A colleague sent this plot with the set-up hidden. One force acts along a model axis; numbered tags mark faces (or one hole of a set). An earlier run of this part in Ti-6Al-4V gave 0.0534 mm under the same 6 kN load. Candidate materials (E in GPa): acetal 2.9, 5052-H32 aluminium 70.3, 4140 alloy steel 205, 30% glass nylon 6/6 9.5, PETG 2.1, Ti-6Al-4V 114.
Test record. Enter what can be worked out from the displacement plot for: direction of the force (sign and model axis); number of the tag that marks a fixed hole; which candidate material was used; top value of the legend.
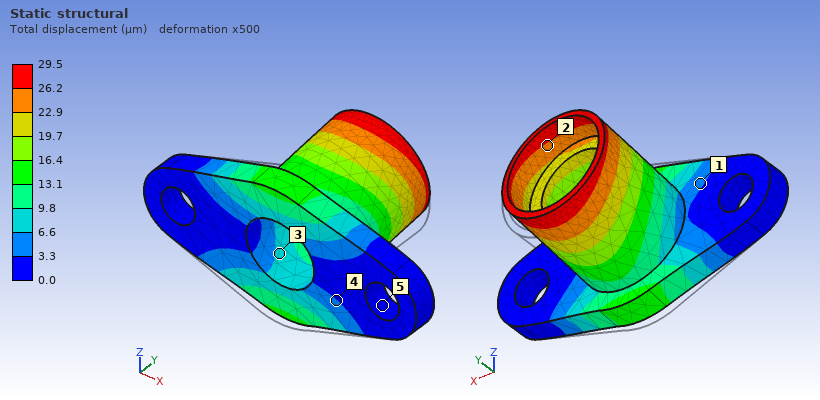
+Z
5
4140 alloy steel
29.5 µm
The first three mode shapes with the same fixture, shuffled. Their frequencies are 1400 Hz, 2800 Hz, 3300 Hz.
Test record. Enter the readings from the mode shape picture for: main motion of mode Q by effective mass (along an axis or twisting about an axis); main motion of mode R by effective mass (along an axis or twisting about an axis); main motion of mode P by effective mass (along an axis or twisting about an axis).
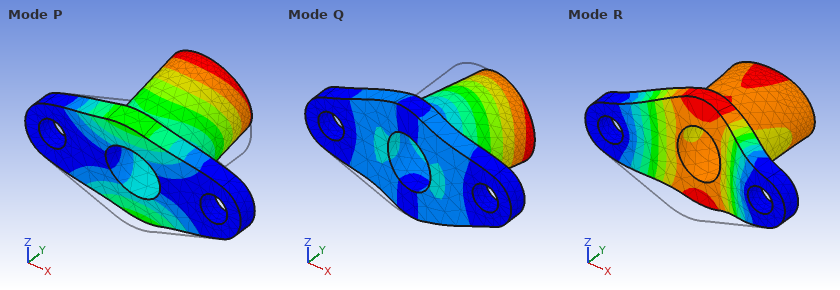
along X
along Y
along Z
